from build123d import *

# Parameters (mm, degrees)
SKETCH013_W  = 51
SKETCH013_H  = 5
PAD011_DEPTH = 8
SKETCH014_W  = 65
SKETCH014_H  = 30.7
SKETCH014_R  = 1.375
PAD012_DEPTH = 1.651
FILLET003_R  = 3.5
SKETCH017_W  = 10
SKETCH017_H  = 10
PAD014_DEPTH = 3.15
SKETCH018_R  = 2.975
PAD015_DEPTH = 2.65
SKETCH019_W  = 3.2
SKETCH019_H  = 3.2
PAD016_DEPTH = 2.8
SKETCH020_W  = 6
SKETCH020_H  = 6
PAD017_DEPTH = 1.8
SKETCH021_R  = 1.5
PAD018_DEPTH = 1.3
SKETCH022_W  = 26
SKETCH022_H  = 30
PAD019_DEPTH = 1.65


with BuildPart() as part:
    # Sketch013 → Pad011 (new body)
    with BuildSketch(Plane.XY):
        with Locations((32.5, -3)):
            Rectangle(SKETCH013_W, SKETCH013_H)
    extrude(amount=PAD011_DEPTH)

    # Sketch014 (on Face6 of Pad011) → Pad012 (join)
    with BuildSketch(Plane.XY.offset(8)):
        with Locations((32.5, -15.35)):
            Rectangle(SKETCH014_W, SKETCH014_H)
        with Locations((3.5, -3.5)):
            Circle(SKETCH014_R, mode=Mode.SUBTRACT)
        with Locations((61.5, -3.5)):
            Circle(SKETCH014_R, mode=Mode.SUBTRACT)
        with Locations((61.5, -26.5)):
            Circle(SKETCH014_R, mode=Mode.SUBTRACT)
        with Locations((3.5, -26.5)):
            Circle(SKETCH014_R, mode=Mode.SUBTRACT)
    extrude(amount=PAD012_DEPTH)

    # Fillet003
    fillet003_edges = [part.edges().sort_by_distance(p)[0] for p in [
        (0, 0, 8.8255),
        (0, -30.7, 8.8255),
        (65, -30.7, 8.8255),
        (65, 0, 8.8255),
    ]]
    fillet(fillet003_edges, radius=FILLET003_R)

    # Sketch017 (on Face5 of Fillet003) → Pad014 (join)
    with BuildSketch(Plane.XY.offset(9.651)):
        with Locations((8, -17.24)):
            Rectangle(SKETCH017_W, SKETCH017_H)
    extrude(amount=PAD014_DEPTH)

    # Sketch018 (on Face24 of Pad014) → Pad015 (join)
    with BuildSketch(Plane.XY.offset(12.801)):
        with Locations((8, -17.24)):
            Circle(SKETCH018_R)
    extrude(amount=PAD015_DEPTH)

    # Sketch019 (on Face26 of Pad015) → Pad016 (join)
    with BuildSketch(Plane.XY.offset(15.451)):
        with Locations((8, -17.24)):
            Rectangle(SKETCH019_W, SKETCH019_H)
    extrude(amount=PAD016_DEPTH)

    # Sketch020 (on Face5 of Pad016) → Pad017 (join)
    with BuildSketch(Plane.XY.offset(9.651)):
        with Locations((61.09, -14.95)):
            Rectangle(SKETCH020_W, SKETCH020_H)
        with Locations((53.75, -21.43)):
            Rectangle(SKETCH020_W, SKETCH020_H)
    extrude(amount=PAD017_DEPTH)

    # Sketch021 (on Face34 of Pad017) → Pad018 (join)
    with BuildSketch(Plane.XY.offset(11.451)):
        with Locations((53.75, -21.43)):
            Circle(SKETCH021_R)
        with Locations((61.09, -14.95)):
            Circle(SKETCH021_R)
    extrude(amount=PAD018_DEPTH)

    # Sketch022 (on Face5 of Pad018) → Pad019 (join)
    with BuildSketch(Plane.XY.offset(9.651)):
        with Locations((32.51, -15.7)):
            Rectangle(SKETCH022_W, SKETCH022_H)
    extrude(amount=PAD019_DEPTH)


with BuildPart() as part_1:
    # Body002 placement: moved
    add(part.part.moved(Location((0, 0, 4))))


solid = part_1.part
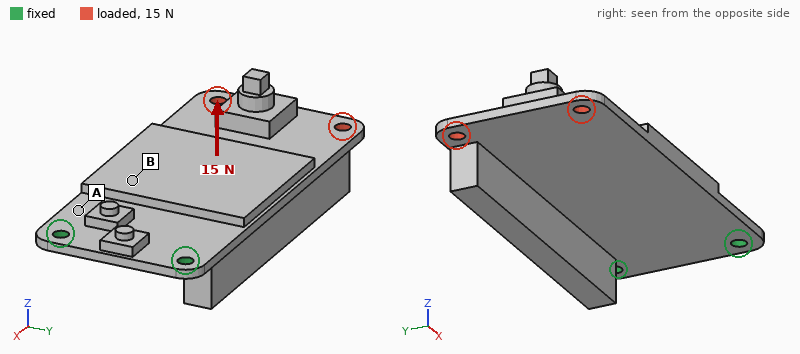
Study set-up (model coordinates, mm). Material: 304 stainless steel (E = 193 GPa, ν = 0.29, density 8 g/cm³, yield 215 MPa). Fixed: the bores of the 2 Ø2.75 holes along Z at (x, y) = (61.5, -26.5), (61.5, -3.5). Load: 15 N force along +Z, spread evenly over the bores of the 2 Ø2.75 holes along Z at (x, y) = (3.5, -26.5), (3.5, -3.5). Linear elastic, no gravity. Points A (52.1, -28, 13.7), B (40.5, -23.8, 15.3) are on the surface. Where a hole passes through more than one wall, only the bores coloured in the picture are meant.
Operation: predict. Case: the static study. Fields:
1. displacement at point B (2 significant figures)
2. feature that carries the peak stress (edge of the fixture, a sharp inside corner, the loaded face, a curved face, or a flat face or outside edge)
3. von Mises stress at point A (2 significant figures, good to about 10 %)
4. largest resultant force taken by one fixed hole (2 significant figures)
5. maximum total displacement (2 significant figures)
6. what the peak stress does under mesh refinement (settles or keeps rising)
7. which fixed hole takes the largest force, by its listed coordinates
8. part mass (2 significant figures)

0.043 mm
edge of the fixture
18 MPa
12 N
0.17 mm
keeps rising
(61.5, -26.5)
57 g
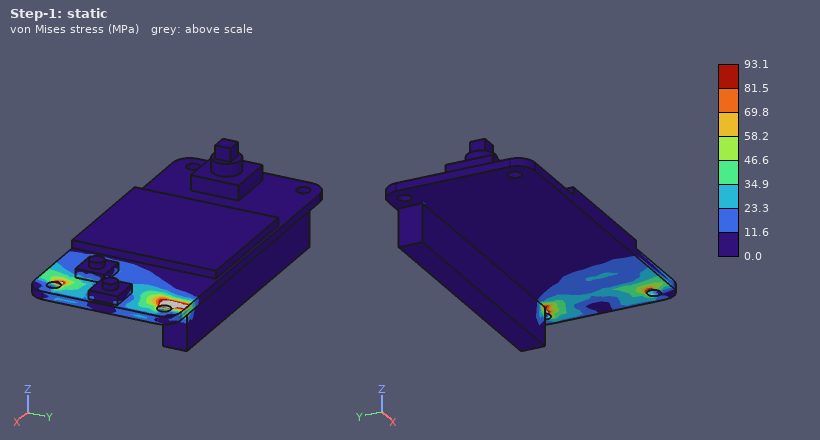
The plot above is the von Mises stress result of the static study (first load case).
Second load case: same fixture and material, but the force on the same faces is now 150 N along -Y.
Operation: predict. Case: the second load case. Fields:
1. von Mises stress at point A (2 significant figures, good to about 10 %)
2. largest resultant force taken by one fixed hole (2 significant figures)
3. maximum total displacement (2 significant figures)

21 MPa
370 N
21 µm
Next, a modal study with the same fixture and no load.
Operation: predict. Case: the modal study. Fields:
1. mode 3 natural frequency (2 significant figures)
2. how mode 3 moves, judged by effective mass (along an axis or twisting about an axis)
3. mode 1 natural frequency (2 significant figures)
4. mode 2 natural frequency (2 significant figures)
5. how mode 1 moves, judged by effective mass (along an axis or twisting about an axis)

4000 Hz
along Y
360 Hz
2200 Hz
along Z
